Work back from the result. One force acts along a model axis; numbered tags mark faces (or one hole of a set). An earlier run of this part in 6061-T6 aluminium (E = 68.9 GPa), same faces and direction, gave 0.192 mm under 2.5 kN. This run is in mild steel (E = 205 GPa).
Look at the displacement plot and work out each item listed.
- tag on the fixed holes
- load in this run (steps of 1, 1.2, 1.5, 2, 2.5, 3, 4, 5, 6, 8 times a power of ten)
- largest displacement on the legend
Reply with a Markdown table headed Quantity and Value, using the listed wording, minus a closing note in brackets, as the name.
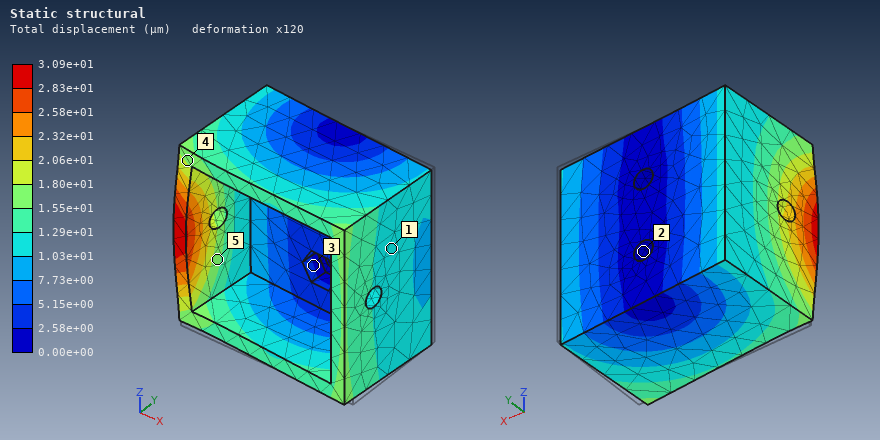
| Quantity | Value |
|---|---|
| tag on the fixed holes | 2 |
| load in this run | 1.2 kN |
| largest displacement on the legend | 3.09e+01 µm |
